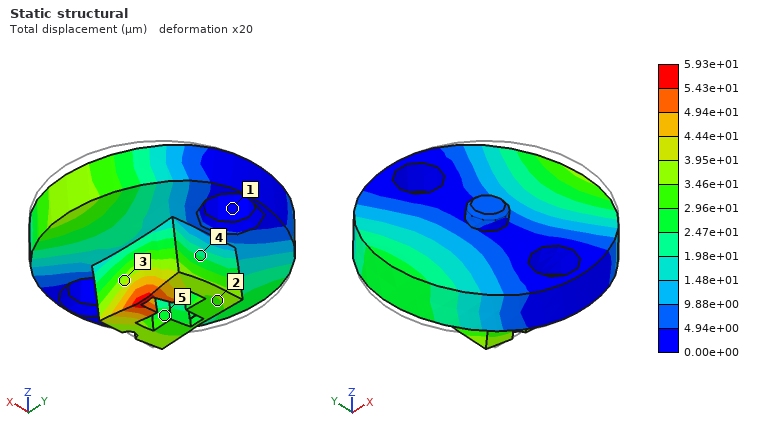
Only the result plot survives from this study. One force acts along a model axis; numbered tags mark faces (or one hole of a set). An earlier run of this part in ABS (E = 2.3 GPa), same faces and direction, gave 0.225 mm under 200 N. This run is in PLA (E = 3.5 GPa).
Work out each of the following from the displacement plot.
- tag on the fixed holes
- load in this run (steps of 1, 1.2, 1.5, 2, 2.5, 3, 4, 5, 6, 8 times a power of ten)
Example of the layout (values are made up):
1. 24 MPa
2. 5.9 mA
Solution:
1. 1
2. 80 N
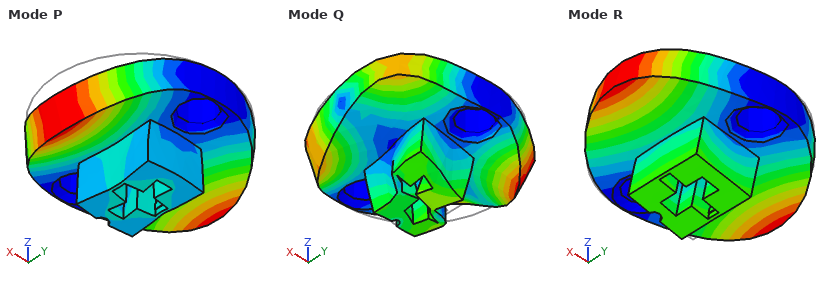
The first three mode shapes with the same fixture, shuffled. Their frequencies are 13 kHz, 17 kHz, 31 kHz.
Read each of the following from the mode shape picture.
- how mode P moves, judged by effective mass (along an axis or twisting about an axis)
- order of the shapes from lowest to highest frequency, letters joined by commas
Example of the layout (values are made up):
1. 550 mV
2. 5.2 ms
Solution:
1. along Z
2. R, P, Q
